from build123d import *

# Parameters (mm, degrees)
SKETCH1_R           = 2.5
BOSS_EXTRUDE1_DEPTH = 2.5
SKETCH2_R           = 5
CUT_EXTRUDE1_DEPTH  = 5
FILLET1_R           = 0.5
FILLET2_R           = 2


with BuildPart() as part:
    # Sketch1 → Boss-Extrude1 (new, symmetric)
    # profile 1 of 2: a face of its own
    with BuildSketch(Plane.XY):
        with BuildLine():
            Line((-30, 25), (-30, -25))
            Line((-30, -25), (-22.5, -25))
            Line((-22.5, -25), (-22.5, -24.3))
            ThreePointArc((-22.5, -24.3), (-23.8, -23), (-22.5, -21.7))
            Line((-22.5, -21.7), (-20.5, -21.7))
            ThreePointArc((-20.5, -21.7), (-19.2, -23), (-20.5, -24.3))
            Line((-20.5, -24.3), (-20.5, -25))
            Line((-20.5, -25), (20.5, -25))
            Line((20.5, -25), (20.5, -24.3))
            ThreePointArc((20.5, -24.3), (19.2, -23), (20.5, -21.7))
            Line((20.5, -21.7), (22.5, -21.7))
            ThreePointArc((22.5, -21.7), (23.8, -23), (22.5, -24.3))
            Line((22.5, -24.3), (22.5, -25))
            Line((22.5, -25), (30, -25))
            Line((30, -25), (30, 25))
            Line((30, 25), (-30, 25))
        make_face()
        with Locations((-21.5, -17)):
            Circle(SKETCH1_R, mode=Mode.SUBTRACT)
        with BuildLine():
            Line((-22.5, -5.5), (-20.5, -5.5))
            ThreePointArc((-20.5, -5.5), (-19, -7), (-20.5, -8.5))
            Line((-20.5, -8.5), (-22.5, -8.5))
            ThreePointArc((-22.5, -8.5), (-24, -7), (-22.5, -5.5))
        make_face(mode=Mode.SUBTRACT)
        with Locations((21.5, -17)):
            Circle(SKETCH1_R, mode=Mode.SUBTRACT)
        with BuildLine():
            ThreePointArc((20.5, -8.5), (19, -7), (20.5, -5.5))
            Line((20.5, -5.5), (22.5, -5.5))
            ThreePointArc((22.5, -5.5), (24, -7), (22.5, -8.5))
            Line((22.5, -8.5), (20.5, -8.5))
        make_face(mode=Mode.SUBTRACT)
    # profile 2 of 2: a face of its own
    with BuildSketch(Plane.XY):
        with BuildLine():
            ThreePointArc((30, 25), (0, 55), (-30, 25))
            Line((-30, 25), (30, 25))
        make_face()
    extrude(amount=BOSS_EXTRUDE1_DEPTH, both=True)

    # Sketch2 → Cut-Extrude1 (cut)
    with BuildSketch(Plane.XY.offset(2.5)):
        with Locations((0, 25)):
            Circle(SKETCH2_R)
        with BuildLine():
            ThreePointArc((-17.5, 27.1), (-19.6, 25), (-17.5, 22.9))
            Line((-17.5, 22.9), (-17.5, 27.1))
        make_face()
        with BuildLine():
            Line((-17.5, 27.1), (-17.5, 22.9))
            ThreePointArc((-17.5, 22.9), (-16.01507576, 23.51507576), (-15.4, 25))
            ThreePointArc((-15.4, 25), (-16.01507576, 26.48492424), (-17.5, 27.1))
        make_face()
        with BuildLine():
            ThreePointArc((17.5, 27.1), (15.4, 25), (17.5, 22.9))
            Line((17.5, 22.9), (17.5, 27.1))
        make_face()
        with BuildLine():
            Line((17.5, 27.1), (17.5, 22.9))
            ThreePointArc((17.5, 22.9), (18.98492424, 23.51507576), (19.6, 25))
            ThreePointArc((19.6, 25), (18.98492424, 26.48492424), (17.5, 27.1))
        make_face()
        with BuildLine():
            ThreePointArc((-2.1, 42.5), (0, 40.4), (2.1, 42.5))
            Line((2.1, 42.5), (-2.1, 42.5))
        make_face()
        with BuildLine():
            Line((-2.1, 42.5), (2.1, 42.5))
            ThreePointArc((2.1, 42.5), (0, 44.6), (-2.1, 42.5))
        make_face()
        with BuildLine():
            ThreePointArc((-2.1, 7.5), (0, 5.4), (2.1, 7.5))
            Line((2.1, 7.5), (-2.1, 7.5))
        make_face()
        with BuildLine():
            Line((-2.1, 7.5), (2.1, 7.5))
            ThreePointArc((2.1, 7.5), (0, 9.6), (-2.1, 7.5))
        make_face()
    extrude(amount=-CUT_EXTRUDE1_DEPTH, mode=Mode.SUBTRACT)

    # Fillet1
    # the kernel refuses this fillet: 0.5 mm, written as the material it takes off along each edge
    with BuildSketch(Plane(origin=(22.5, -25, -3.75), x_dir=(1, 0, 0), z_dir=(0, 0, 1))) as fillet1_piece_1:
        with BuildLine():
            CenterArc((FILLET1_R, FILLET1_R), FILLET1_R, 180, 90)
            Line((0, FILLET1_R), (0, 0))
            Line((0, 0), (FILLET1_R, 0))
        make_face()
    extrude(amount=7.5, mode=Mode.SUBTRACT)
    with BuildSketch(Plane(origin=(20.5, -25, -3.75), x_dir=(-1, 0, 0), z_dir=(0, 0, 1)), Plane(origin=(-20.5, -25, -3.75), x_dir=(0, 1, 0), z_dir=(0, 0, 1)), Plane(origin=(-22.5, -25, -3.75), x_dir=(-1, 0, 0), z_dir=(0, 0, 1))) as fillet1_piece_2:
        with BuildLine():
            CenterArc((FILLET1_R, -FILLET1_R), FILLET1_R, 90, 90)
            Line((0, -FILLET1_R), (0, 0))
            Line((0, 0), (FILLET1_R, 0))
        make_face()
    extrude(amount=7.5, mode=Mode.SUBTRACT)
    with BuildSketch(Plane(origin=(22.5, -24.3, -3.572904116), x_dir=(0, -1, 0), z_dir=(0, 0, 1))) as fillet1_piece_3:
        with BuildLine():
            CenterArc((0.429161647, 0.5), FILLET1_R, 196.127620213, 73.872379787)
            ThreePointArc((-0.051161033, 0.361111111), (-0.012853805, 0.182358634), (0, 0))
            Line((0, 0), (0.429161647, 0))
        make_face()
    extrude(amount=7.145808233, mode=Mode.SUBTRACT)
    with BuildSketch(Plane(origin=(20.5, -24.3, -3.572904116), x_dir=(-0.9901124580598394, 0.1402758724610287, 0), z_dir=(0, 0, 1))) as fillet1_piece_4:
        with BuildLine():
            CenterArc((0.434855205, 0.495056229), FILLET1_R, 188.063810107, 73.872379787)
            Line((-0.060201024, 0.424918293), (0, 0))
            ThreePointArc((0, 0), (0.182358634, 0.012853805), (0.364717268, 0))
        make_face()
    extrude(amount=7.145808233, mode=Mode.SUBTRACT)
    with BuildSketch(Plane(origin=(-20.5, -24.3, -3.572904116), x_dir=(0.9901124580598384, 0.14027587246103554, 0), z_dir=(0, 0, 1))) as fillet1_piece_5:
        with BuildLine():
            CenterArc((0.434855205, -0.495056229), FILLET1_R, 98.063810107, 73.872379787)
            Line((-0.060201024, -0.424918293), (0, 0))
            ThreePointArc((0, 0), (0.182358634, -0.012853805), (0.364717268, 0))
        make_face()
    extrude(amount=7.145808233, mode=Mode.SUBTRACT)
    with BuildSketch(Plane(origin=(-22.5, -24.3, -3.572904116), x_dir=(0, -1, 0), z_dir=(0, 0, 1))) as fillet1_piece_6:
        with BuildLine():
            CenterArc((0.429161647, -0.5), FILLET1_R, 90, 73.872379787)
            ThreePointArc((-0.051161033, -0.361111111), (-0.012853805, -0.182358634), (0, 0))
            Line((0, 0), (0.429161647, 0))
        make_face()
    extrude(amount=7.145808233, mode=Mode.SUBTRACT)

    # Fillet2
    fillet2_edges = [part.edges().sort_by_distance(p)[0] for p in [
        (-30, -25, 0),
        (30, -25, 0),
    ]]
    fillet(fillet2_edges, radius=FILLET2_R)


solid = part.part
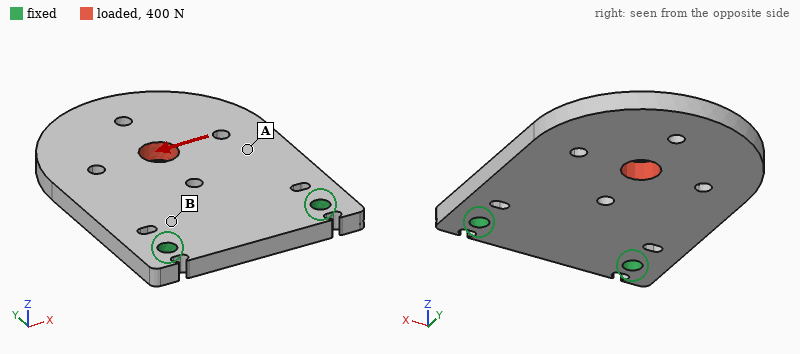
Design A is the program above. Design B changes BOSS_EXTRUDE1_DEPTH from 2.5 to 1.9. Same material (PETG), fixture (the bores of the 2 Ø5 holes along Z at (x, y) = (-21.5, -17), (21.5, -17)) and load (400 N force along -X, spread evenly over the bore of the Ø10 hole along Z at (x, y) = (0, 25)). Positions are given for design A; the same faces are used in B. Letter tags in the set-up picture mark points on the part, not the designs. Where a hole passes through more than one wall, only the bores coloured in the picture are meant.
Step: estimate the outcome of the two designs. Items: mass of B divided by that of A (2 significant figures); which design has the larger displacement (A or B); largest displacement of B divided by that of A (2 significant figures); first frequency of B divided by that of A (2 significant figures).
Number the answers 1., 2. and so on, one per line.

1. 0.76
2. B
3. 1.3
4. 0.77
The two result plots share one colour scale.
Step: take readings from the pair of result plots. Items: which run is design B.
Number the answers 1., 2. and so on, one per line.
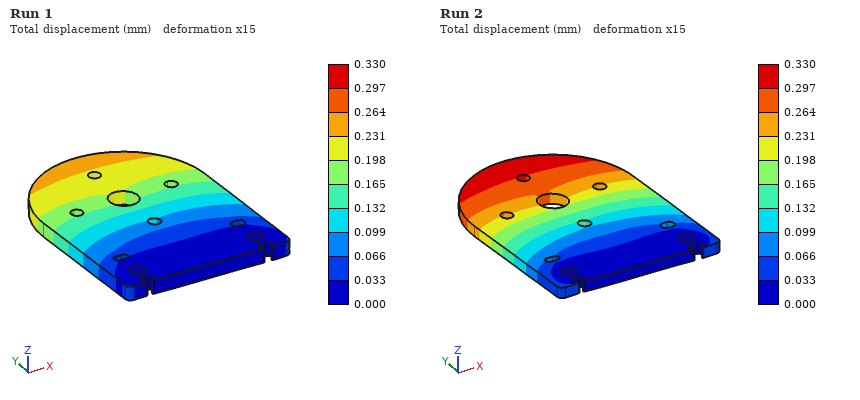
1. Run 2
